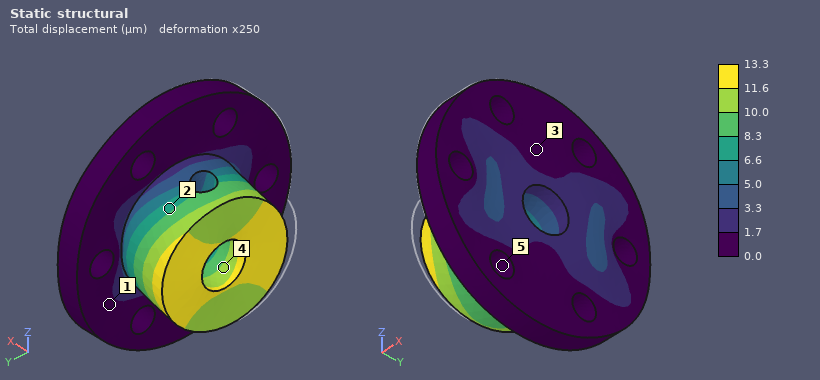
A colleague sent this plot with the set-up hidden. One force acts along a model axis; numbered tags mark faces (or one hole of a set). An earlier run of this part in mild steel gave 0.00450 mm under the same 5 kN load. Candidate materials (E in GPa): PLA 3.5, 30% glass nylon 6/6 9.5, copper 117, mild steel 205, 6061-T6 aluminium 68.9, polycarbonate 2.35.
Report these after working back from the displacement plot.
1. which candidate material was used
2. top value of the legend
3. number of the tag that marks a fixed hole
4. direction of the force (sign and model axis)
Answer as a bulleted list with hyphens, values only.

- 6061-T6 aluminium
- 13.3 µm
- 5
- +Y
